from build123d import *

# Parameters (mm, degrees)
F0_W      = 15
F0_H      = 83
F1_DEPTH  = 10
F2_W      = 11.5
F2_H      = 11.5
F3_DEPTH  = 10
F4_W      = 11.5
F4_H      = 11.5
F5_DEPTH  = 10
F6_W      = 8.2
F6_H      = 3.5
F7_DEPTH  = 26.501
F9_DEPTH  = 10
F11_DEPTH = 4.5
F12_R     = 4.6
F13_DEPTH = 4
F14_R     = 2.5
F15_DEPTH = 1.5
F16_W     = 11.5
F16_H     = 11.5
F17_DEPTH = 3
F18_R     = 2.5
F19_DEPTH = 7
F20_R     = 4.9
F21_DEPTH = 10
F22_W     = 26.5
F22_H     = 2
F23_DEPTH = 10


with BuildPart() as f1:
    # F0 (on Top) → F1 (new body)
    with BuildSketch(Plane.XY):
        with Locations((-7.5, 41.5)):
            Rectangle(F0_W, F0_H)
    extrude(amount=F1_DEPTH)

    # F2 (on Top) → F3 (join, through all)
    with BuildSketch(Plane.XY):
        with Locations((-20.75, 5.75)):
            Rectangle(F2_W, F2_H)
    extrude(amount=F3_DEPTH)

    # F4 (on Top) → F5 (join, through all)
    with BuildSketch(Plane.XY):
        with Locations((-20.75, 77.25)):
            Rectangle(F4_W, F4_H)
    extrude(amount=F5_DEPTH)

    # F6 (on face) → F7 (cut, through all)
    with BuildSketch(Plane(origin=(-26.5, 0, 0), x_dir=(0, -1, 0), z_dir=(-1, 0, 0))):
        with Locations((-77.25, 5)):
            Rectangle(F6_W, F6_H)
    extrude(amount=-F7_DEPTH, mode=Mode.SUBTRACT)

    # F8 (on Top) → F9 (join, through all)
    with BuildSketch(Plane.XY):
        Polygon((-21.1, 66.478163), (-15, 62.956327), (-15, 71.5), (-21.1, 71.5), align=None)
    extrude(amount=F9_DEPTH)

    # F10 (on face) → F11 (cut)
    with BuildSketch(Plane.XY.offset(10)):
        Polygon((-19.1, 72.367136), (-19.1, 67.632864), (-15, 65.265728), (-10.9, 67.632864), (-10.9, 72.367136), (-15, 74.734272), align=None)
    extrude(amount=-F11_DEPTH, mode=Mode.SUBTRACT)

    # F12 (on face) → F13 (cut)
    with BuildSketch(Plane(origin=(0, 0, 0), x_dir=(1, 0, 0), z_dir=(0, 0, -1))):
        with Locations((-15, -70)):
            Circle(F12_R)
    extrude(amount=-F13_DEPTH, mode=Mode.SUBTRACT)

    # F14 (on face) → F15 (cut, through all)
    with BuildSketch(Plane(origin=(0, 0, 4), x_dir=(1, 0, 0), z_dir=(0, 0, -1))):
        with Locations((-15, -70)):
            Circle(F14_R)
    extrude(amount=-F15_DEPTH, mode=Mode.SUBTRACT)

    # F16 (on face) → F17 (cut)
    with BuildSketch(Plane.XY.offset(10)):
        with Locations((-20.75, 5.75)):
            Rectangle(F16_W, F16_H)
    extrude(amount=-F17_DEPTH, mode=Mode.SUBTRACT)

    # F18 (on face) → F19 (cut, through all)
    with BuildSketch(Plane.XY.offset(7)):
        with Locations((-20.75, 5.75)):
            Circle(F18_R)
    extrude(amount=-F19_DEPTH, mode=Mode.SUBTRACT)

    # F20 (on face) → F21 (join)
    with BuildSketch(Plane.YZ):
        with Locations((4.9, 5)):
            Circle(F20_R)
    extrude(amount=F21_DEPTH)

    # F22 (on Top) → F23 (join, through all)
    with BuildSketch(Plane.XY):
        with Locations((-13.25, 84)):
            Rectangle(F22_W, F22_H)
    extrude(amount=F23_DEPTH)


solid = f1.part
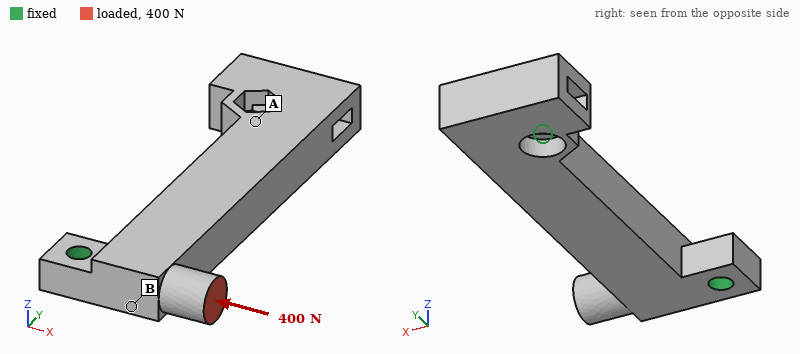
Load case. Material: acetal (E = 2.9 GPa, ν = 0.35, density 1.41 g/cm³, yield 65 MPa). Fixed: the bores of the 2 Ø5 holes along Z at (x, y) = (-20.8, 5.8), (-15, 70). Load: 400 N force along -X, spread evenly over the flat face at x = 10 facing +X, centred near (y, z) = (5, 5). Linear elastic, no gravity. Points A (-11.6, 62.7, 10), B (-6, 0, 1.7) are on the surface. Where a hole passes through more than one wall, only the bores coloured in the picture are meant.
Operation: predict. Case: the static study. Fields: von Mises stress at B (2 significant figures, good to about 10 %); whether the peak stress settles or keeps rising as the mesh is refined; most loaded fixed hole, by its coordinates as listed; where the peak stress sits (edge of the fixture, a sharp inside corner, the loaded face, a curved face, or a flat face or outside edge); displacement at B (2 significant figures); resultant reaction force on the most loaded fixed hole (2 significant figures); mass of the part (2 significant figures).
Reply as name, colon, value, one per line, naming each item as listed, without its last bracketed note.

von Mises stress at B: 4.7 MPa
whether the peak stress settles or keeps rising as the mesh is refined: keeps rising
most loaded fixed hole, by its coordinates as listed: (-20.8, 5.8)
where the peak stress sits: edge of the fixture
displacement at B: 0.042 mm
resultant reaction force on the most loaded fixed hole: 400 N
mass of the part: 21 g
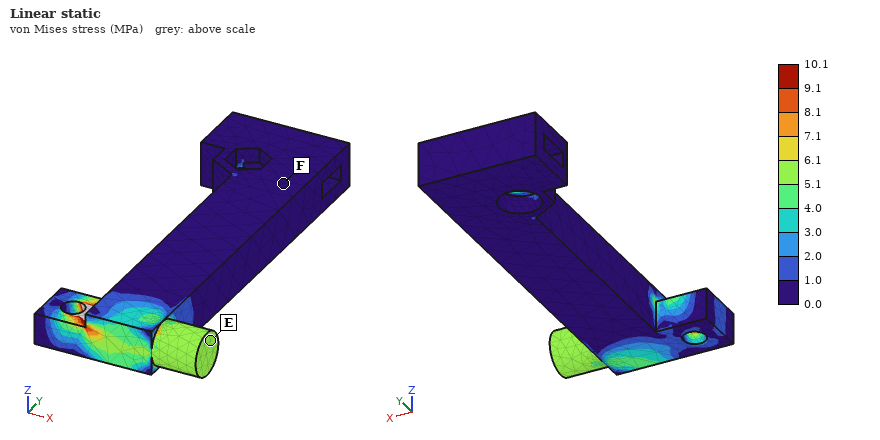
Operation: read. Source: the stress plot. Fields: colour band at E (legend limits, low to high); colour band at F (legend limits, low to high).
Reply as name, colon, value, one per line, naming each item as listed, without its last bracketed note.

colour band at E: 5.1 to 6.1 MPa
colour band at F: 0.0 to 1.0 MPa
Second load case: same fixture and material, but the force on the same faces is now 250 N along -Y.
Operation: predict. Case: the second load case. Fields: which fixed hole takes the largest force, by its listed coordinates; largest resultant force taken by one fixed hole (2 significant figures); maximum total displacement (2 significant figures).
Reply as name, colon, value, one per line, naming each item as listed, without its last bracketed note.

which fixed hole takes the largest force, by its listed coordinates: (-15, 70)
largest resultant force taken by one fixed hole: 250 N
maximum total displacement: 0.36 mm
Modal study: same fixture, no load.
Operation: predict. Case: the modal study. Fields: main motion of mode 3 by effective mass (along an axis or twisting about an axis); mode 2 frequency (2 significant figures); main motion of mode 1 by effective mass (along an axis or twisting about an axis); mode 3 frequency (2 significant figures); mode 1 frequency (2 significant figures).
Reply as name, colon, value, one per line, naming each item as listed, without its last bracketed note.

main motion of mode 3 by effective mass: twisting about X
mode 2 frequency: 2000 Hz
main motion of mode 1 by effective mass: along Z
mode 3 frequency: 2400 Hz
mode 1 frequency: 1200 Hz
